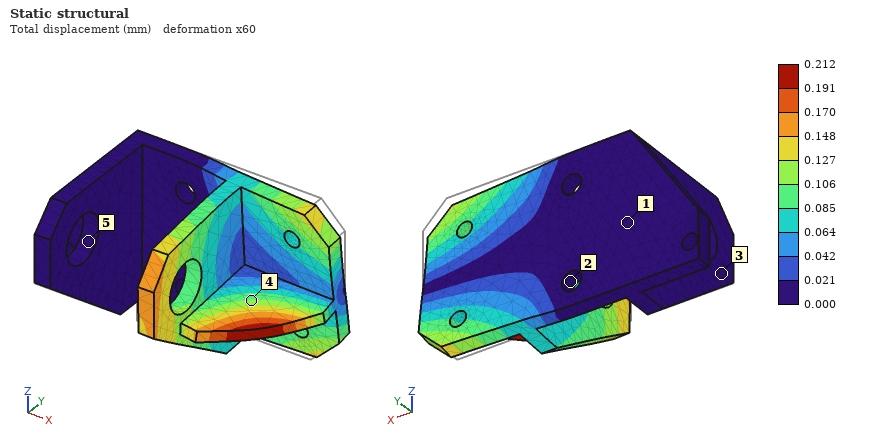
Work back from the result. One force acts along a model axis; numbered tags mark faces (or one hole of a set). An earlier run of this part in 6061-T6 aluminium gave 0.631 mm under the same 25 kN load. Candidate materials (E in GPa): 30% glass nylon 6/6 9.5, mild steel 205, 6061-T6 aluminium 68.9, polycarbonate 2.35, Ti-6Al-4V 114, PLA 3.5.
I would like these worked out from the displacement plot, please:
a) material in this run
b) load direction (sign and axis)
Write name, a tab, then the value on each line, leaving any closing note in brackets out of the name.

material in this run	mild steel
load direction	-Z
